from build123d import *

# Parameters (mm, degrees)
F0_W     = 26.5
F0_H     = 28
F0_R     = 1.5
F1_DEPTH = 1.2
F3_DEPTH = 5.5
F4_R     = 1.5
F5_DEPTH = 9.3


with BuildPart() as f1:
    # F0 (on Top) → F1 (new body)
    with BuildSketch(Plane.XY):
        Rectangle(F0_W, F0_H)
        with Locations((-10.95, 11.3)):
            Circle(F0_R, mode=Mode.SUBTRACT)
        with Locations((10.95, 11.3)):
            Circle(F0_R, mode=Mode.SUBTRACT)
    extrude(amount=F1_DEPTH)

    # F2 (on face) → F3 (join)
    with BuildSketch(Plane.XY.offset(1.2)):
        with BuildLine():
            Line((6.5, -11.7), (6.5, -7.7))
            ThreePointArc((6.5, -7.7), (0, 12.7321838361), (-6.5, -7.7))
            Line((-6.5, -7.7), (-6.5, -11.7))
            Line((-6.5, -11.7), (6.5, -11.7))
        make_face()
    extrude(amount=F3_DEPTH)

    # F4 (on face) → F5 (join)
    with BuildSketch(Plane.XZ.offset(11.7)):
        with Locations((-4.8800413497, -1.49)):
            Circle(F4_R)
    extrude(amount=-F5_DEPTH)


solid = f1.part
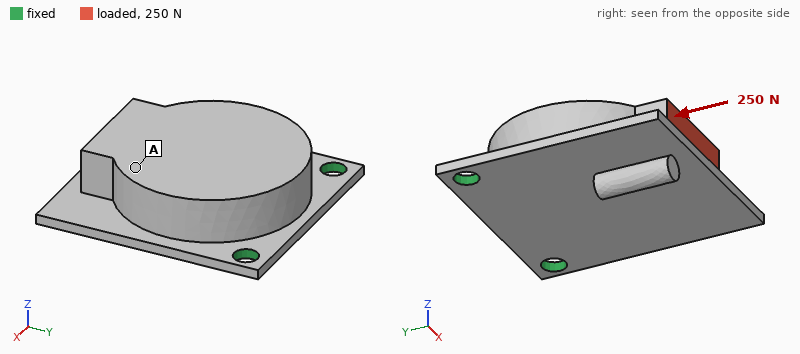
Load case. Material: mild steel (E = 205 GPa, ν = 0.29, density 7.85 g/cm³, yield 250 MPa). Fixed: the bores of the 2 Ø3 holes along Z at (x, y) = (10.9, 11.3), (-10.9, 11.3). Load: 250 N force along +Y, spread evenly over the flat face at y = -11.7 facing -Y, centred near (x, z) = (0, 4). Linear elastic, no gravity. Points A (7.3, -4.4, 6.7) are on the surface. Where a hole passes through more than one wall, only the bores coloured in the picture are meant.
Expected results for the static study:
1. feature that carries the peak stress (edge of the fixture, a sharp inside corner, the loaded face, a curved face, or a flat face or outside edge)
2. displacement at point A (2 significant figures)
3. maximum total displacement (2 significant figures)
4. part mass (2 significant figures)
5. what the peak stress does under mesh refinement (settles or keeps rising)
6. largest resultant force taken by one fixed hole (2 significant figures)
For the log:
edge of the fixture
39 µm
60 µm
26 g
keeps rising
130 N
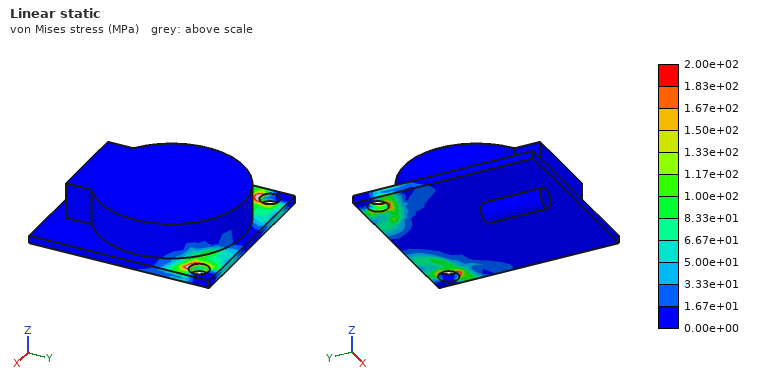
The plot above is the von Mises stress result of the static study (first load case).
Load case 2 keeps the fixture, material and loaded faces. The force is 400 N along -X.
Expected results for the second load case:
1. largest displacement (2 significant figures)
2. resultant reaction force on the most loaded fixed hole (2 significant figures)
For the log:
5.4 µm
470 N
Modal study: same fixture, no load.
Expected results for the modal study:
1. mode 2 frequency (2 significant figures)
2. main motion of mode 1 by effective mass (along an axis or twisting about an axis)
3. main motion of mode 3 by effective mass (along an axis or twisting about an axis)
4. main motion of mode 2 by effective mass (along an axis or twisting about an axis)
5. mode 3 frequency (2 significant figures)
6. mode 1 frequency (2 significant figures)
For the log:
13 kHz
along Z
along X
twisting about Y
15 kHz
1500 Hz
